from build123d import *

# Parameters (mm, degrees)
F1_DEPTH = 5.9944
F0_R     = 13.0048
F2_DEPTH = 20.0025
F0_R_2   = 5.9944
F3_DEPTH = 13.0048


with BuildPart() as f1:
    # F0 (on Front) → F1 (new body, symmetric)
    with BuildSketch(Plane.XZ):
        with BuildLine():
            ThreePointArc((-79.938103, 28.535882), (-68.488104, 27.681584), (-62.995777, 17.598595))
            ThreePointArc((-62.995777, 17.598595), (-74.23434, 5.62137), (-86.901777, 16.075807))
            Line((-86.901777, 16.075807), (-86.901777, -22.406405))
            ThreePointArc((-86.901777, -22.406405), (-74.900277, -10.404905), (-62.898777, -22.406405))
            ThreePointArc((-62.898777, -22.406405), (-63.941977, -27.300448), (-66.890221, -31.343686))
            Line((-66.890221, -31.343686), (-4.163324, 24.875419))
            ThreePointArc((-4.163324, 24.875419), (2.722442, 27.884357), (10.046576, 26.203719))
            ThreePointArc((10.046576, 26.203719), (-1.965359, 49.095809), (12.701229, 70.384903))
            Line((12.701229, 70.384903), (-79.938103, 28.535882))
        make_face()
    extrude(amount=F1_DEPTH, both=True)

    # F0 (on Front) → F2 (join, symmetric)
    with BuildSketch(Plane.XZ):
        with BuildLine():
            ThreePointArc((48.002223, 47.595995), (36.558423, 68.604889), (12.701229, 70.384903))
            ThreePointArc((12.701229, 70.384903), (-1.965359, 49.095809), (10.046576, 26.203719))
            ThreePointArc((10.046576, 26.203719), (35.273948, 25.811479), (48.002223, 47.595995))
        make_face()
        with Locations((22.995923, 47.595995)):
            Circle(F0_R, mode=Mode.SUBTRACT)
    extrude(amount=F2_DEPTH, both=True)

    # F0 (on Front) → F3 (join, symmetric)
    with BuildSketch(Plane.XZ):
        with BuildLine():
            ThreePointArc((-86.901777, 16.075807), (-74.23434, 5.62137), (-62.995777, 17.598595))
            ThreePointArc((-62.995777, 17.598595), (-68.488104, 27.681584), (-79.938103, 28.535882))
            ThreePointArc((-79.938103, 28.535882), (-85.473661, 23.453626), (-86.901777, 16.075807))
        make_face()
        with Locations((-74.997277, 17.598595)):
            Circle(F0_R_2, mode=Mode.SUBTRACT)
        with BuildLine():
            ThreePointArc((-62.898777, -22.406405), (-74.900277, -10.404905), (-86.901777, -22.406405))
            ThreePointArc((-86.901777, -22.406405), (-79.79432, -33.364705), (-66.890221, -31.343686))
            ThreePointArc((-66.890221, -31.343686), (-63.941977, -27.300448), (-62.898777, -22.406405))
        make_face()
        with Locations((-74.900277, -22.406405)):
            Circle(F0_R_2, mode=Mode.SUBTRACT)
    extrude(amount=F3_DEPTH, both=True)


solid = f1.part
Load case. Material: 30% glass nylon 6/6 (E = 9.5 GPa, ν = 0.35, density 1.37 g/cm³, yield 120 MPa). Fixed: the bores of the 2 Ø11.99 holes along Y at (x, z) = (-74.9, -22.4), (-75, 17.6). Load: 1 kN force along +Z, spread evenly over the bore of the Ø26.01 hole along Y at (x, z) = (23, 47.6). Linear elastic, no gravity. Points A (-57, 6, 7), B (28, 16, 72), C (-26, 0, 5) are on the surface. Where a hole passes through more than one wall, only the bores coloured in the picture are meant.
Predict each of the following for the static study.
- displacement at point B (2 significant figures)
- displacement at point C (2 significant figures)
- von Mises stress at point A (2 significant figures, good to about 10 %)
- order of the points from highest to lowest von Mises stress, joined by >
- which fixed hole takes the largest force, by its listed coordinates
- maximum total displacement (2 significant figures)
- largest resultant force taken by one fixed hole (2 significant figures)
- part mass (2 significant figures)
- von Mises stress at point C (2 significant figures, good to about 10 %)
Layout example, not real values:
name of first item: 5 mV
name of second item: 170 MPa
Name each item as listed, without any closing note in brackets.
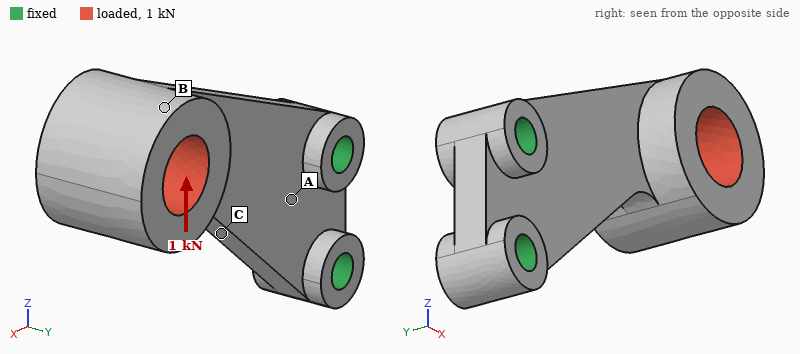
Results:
displacement at point B: 0.55 mm
displacement at point C: 0.093 mm
von Mises stress at point A: 4.7 MPa
order of the points from highest to lowest von Mises stress, joined by >: C > A > B
which fixed hole takes the largest force, by its listed coordinates: (-74.9, -22.4)
maximum total displacement: 0.61 mm
largest resultant force taken by one fixed hole: 2.4 kN
part mass: 160 g
von Mises stress at point C: 17 MPa
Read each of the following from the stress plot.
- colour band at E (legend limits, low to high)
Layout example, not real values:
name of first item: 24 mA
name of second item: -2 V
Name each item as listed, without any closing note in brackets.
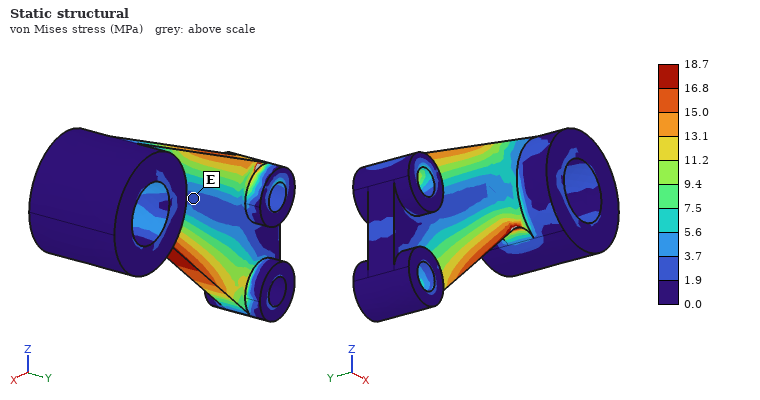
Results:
colour band at E: 1.9 to 3.7 MPa
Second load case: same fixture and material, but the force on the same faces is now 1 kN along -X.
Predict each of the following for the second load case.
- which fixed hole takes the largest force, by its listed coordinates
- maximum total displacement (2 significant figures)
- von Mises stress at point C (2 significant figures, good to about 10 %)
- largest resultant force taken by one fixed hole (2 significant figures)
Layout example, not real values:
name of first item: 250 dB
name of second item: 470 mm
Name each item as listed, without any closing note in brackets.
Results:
which fixed hole takes the largest force, by its listed coordinates: (-75, 17.6)
maximum total displacement: 0.21 mm
von Mises stress at point C: 5.0 MPa
largest resultant force taken by one fixed hole: 1.6 kN
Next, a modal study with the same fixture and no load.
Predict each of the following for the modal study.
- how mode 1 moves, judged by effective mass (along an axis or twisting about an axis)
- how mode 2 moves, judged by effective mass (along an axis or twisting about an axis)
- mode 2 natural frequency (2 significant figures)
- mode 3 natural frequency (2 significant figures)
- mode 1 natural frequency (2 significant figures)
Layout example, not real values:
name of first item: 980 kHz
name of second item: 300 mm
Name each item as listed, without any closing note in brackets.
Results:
how mode 1 moves, judged by effective mass: along Y
how mode 2 moves, judged by effective mass: along Z
mode 2 natural frequency: 770 Hz
mode 3 natural frequency: 940 Hz
mode 1 natural frequency: 240 Hz
